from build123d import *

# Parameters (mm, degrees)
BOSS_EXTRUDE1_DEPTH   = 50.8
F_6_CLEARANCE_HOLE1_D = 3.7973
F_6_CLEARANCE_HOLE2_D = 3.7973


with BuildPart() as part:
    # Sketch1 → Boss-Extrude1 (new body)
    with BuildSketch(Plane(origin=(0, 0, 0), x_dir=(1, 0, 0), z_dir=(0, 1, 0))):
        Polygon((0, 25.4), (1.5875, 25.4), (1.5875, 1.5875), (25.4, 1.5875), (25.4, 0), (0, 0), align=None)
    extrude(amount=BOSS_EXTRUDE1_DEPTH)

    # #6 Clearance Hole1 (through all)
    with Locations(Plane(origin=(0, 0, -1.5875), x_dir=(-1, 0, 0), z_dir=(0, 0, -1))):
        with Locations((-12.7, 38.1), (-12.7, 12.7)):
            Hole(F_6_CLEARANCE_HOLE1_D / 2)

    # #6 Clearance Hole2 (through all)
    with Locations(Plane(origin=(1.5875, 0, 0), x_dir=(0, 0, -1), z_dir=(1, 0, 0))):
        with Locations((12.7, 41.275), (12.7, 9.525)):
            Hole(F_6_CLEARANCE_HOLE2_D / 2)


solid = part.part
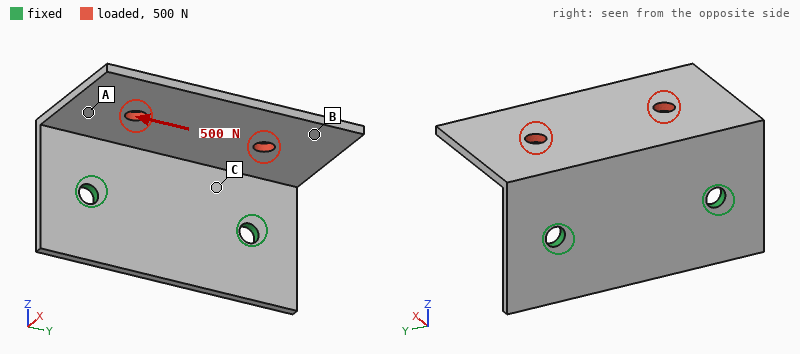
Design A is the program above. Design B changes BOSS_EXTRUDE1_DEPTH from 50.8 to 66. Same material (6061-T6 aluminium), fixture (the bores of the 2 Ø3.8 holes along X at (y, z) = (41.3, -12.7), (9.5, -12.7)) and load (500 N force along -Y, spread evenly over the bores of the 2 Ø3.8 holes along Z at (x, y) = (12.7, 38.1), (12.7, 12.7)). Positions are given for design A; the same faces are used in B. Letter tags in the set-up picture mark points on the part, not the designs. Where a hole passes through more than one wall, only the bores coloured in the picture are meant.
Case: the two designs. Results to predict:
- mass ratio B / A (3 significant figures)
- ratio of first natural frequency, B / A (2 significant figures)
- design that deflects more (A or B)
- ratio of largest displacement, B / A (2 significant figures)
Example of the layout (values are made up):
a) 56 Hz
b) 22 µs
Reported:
a) 1.30
b) 0.94
c) B
d) 1.2
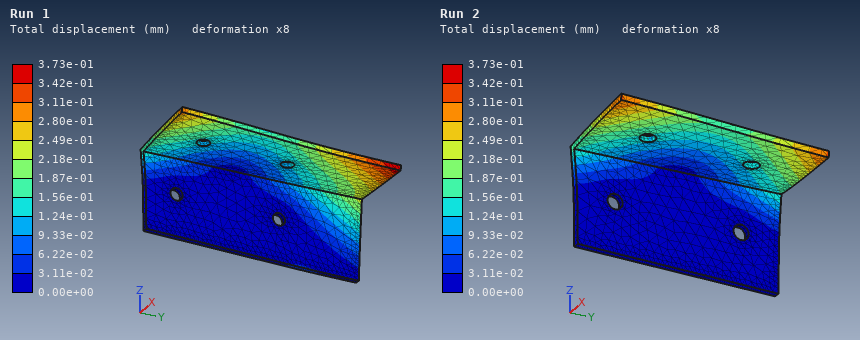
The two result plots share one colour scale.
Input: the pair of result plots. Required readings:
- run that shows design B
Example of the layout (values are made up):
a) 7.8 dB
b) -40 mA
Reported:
a) Run 1
